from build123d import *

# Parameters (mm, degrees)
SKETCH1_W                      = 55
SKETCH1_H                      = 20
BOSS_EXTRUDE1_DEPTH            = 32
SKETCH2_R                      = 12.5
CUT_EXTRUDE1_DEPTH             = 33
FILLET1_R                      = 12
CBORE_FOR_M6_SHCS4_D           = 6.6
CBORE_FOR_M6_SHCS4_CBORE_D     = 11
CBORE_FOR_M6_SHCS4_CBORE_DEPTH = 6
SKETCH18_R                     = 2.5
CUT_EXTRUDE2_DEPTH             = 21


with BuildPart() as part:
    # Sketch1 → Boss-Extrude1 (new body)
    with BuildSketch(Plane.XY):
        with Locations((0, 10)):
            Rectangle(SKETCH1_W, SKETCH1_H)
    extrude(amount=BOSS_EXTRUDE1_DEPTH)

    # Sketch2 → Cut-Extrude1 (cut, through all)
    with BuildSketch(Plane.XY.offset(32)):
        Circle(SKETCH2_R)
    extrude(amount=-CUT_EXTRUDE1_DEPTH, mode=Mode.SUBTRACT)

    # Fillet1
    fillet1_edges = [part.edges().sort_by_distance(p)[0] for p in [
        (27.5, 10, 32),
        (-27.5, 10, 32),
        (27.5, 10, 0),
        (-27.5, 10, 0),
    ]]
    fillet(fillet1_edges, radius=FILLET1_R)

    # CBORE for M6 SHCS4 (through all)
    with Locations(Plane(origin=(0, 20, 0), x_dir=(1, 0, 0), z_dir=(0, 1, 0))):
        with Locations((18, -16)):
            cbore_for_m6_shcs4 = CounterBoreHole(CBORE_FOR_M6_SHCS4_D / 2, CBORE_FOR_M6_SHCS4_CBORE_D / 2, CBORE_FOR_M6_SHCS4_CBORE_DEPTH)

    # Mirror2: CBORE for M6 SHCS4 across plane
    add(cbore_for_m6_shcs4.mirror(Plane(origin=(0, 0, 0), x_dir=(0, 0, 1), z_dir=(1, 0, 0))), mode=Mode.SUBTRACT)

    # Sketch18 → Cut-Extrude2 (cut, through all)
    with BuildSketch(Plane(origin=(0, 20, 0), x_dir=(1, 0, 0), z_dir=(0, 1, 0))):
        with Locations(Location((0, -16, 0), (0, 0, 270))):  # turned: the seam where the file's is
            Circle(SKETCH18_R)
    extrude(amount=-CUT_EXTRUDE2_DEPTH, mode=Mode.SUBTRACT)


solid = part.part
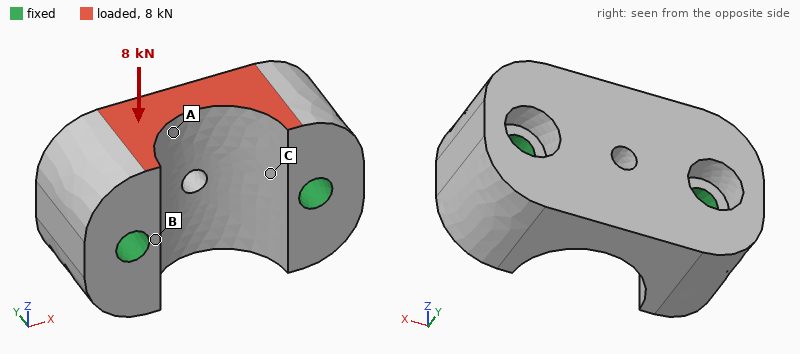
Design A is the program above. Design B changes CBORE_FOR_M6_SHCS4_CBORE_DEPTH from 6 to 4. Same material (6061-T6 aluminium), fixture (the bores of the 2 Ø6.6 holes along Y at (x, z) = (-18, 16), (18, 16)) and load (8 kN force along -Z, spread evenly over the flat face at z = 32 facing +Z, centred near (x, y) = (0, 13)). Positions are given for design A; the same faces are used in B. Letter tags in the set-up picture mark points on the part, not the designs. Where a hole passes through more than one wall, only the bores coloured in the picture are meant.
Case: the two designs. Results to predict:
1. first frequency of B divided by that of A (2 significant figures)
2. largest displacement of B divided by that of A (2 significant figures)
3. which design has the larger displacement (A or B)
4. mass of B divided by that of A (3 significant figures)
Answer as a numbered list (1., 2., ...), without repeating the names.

1. 1.2
2. 0.79
3. A
4. 1.01
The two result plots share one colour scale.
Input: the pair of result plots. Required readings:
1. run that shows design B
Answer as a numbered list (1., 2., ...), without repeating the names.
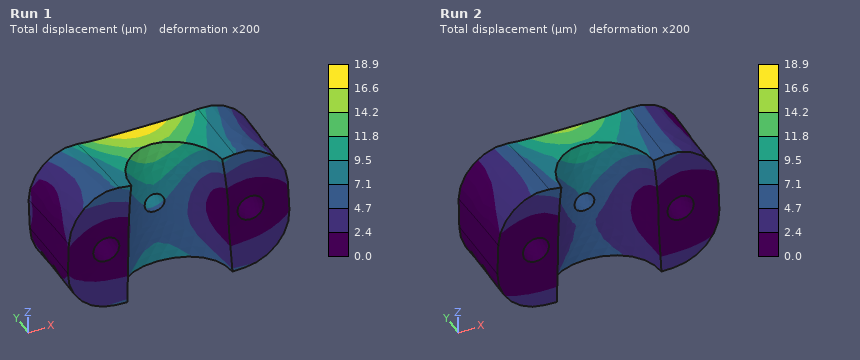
1. Run 2
